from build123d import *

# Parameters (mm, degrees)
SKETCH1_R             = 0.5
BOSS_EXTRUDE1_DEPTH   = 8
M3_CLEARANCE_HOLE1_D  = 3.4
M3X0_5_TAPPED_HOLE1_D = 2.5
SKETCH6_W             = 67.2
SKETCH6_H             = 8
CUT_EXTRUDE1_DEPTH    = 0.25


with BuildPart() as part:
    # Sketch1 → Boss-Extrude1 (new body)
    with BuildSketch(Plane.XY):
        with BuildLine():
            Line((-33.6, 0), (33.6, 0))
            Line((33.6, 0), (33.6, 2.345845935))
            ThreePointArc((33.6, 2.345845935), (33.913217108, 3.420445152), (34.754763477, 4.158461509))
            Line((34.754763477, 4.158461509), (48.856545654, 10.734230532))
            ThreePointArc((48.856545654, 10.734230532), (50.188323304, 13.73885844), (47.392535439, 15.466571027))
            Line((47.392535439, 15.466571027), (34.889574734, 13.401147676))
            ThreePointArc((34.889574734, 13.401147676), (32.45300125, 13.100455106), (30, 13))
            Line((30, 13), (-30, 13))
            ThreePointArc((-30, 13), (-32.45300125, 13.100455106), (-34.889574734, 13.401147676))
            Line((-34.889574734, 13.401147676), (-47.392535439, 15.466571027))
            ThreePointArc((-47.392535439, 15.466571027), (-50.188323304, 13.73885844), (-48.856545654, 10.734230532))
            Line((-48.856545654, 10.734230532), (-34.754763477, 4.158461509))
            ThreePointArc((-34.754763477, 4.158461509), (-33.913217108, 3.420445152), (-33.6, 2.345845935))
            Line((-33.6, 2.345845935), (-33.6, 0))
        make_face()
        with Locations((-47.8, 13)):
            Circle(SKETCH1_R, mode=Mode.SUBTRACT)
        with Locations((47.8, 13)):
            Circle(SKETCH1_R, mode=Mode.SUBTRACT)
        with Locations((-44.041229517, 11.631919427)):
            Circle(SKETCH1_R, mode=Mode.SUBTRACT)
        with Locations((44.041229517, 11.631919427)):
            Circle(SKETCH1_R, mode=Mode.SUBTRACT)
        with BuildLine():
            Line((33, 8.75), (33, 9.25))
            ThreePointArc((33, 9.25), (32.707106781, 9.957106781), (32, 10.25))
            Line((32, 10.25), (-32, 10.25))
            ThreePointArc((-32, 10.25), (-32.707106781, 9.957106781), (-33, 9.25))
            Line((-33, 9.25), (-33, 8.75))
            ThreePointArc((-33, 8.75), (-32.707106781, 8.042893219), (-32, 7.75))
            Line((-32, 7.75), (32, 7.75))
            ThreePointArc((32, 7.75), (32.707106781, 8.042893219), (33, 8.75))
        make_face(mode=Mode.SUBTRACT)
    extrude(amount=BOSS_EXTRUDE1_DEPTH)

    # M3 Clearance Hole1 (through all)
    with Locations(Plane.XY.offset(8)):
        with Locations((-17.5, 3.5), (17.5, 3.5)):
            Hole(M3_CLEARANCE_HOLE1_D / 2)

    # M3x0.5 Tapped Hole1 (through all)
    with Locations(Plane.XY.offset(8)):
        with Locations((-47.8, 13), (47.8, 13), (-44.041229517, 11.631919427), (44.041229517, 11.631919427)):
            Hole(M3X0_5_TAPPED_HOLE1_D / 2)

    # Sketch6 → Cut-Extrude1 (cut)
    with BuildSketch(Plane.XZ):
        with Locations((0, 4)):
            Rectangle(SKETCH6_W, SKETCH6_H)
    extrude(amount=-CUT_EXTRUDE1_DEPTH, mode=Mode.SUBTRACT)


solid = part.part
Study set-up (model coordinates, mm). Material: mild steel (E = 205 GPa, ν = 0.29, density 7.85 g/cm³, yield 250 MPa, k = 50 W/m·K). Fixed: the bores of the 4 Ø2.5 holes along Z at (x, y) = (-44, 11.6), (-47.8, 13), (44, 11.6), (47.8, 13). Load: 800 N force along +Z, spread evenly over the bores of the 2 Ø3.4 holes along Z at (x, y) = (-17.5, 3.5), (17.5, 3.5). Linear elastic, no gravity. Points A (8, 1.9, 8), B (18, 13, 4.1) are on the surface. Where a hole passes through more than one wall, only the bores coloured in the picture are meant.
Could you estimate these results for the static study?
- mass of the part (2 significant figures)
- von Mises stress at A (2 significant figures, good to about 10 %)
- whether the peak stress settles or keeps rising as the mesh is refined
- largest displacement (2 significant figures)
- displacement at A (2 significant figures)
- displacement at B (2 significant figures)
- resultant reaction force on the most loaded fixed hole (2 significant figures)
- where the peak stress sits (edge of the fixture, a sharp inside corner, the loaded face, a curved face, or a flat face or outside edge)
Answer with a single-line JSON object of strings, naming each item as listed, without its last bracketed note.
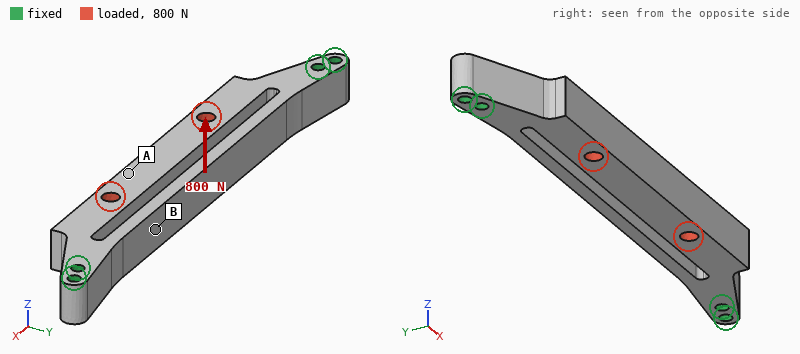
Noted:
{"mass of the part": "56 g", "von Mises stress at A": "42 MPa", "whether the peak stress settles or keeps rising as the mesh is refined": "keeps rising", "largest displacement": "41 µm", "displacement at A": "39 µm", "displacement at B": "11 µm", "resultant reaction force on the most loaded fixed hole": "480 N", "where the peak stress sits": "edge of the fixture"}
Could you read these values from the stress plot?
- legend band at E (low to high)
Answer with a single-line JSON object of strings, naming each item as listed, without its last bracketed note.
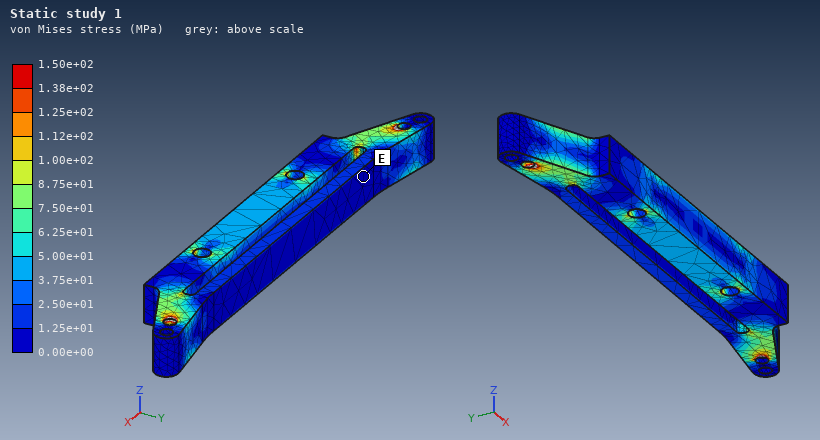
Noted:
{"legend band at E": "0.00e+00 to 1.25e+01 MPa"}
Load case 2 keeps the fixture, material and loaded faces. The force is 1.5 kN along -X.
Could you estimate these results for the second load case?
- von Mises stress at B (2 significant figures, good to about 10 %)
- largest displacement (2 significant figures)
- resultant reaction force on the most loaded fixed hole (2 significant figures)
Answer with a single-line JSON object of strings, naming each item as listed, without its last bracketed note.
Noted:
{"von Mises stress at B": "7.7 MPa", "largest displacement": "7.0 µm", "resultant reaction force on the most loaded fixed hole": "790 N"}
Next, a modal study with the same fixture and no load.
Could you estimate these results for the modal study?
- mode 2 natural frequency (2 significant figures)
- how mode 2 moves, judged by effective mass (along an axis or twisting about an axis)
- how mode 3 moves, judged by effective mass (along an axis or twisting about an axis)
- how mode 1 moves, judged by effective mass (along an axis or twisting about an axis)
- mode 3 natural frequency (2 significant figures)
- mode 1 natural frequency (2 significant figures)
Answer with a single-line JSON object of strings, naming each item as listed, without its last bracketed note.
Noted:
{"mode 2 natural frequency": "4500 Hz", "how mode 2 moves, judged by effective mass": "along Z", "how mode 3 moves, judged by effective mass": "along Y", "how mode 1 moves, judged by effective mass": "along Y", "mode 3 natural frequency": "5400 Hz", "mode 1 natural frequency": "3100 Hz"}
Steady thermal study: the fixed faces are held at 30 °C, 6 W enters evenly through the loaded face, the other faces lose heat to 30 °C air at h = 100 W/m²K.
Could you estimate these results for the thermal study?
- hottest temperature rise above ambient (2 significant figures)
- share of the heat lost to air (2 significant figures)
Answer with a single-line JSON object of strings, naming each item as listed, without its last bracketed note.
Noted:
{"hottest temperature rise above ambient": "18 K", "share of the heat lost to air": "56 %"}
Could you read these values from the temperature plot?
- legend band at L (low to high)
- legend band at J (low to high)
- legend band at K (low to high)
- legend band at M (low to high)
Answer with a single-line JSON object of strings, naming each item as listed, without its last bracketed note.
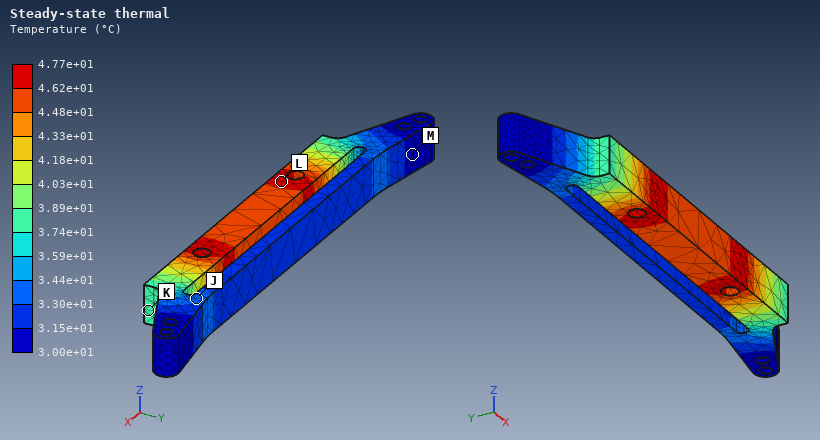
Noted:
{"legend band at L": "4.62e+01 to 4.77e+01 °C", "legend band at J": "3.30e+01 to 3.44e+01 °C", "legend band at K": "3.74e+01 to 3.89e+01 °C", "legend band at M": "3.00e+01 to 3.15e+01 °C"}
